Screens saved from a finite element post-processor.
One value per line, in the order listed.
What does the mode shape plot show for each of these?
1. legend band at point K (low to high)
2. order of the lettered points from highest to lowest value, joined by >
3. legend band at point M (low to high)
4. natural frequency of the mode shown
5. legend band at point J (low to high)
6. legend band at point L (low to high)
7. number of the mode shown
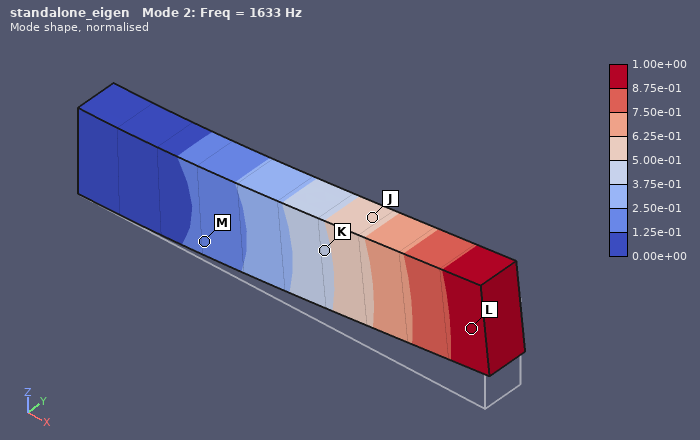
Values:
3.75e-01 to 5.00e-01
L > J > K > M
1.25e-01 to 2.50e-01
1633 Hz
5.00e-01 to 6.25e-01
8.75e-01 to 1.00e+00
2
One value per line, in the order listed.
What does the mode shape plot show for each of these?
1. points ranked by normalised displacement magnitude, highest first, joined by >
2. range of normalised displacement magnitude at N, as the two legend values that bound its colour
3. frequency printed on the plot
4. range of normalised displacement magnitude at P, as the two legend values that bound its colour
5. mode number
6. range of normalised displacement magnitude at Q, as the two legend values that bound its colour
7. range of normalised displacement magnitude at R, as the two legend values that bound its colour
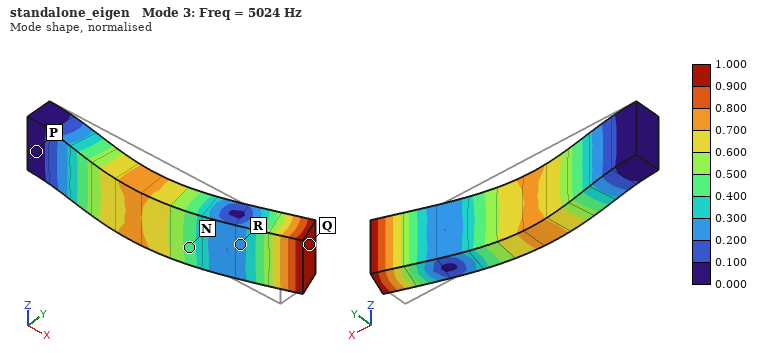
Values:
Q > N > R > P
0.400 to 0.500
5024 Hz
0.000 to 0.100
3
0.900 to 1.000
0.200 to 0.300
